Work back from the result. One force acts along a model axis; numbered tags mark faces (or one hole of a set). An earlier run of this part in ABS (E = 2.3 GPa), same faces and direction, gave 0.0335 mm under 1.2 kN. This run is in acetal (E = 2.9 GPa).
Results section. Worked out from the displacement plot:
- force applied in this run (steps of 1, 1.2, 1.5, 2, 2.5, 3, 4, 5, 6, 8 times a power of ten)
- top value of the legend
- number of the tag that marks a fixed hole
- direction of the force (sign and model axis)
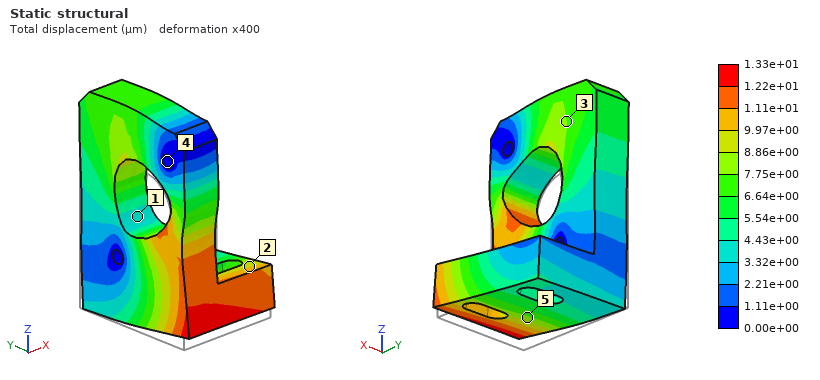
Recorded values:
600 N
1.33e+01 µm
4
+Z
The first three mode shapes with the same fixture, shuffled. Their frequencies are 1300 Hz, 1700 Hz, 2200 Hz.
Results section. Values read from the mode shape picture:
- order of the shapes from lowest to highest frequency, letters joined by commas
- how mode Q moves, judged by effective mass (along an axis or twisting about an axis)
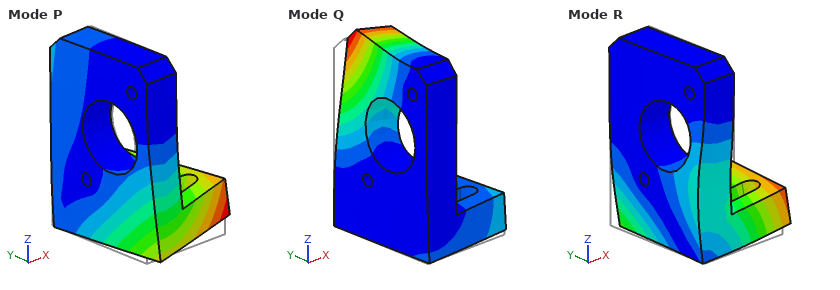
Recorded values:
P, R, Q
along X
